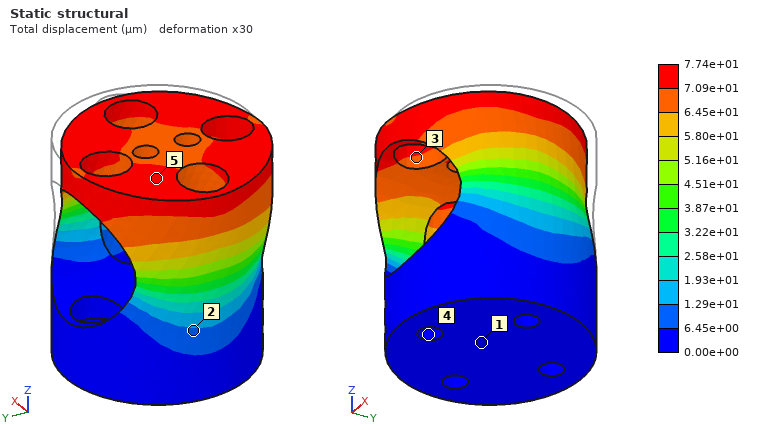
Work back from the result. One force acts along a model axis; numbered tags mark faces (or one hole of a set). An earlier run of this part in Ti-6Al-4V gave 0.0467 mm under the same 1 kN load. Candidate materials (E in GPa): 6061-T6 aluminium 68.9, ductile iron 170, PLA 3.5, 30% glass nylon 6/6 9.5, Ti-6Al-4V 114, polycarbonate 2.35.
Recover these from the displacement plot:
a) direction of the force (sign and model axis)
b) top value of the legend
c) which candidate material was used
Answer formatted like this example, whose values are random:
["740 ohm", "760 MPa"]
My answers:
["-X", "7.74e+01 µm", "6061-T6 aluminium"]
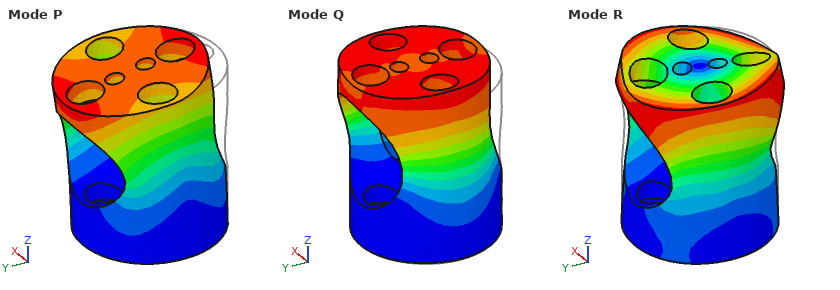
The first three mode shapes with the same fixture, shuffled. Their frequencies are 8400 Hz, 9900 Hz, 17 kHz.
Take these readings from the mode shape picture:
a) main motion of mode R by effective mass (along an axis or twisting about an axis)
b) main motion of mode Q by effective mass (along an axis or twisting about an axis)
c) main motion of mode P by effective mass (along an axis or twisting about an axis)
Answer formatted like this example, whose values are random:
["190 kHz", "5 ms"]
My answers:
["twisting about Z", "along X", "along Y"]
